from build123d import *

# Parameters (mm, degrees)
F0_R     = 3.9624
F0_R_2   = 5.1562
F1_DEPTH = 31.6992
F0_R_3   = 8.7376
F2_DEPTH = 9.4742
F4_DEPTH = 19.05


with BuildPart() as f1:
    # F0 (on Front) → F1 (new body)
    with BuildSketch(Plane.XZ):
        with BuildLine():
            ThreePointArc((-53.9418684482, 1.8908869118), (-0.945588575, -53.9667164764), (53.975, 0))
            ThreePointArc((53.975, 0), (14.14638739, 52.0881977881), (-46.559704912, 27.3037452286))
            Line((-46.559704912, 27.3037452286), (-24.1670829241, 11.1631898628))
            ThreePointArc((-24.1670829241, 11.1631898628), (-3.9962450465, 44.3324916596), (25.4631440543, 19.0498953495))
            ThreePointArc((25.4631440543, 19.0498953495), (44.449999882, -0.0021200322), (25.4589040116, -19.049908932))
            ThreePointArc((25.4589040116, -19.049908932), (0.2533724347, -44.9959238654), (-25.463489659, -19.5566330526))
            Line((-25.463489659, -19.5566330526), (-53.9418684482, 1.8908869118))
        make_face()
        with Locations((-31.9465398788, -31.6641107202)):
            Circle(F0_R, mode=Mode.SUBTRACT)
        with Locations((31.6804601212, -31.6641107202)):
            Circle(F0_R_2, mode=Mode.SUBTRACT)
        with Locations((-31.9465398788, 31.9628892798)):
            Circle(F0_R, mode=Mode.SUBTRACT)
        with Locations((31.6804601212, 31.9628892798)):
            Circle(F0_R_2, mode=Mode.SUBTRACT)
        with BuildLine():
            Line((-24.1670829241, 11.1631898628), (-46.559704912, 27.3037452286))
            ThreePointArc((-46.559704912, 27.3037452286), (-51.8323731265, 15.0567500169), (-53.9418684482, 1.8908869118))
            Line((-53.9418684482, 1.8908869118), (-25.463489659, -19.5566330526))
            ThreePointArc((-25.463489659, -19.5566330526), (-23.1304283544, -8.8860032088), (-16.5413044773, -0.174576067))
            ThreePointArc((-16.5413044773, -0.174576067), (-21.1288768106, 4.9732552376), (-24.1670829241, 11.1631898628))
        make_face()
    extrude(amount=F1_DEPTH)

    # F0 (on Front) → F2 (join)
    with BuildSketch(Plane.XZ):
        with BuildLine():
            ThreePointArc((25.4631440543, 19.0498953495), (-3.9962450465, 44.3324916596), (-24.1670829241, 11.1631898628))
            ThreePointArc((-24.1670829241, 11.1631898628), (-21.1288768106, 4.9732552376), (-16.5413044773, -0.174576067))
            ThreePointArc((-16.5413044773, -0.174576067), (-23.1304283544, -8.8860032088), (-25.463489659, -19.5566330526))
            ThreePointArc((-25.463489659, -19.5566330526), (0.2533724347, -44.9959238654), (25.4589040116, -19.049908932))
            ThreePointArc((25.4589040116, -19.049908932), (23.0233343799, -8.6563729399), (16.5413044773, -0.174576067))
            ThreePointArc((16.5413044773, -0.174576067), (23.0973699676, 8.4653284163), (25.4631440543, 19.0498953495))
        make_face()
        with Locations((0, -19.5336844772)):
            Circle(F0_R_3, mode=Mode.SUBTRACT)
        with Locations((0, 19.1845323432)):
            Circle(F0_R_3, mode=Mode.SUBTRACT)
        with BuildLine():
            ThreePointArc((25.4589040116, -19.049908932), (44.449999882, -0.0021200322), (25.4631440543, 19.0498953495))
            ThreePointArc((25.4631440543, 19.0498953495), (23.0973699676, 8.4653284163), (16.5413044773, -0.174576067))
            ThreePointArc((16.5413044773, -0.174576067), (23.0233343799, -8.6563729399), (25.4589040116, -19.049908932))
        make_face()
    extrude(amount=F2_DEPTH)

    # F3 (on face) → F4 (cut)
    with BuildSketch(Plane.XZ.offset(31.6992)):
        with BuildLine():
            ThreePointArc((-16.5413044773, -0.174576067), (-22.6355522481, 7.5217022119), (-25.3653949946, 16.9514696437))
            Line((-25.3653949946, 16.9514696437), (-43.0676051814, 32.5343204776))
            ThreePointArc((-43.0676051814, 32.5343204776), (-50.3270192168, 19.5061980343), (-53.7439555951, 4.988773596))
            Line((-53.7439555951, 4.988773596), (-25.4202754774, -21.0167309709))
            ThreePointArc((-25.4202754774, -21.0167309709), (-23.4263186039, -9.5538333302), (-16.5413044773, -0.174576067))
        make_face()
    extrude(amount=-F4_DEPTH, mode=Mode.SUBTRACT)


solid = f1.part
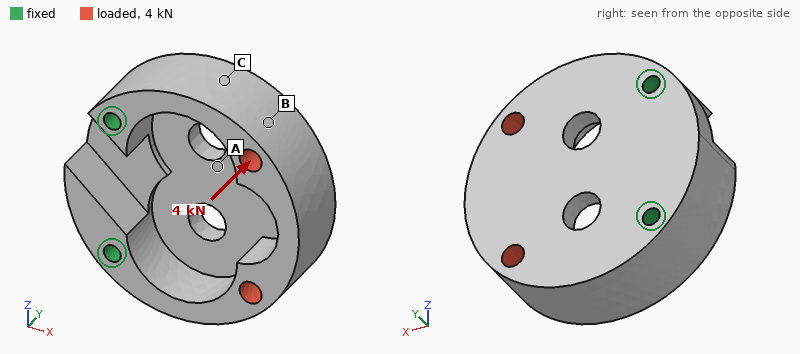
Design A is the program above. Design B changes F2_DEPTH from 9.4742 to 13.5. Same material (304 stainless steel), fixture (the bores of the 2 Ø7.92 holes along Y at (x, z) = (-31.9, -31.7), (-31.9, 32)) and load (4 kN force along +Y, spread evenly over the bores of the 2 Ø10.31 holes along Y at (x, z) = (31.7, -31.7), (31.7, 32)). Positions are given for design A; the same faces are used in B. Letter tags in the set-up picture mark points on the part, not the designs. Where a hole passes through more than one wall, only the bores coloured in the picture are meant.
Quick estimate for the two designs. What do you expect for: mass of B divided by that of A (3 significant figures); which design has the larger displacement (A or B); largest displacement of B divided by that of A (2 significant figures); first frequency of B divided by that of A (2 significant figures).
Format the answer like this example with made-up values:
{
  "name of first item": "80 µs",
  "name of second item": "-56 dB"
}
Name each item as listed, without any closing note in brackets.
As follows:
{
  "mass of B divided by that of A": "1.10",
  "which design has the larger displacement": "A",
  "largest displacement of B divided by that of A": "0.85",
  "first frequency of B divided by that of A": "1.0"
}
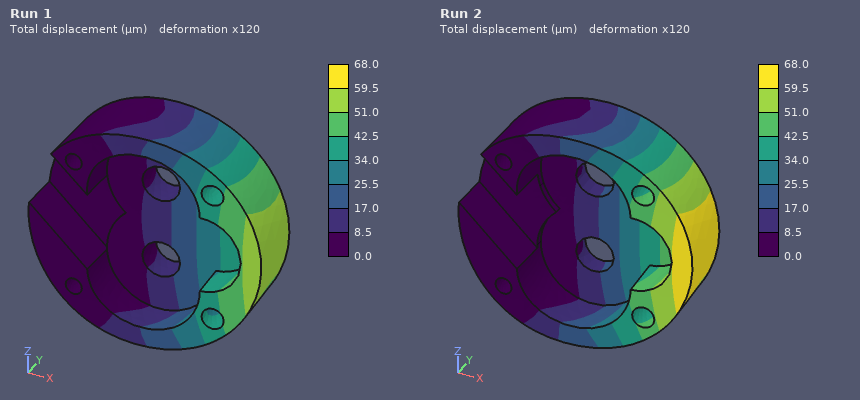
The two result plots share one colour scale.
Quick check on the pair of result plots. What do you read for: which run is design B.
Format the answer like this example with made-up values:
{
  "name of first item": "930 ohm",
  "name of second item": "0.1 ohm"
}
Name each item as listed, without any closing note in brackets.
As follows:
{
  "which run is design B": "Run 1"
}
